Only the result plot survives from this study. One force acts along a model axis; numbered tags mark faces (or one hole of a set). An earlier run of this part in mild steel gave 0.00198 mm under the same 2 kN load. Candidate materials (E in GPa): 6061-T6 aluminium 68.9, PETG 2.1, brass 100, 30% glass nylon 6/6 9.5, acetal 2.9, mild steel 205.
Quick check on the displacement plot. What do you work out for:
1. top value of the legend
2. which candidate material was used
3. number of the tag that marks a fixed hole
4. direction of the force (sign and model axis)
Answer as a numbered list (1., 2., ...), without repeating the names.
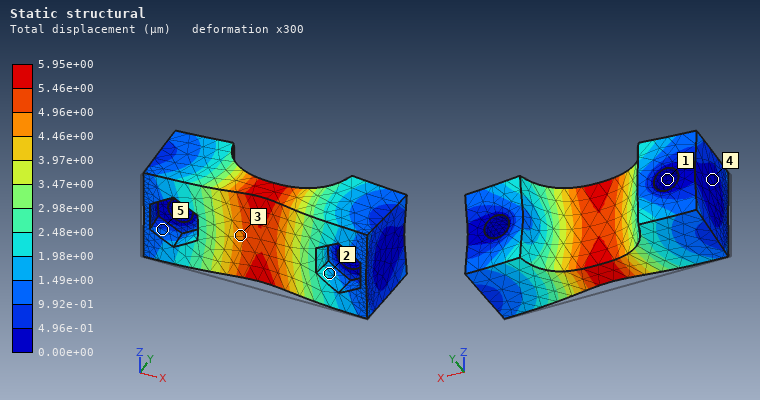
1. 5.95e+00 µm
2. 6061-T6 aluminium
3. 1
4. +Y
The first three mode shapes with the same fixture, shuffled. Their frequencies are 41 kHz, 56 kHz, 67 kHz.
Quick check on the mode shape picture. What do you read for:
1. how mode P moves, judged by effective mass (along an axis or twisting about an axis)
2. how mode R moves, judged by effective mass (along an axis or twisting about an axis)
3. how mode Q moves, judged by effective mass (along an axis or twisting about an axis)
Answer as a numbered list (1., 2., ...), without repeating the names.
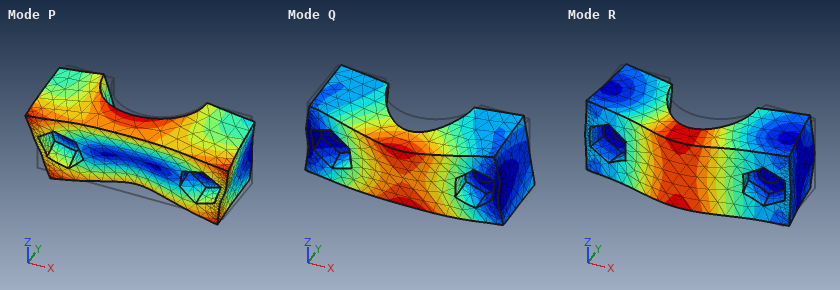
1. twisting about X
2. along Y
3. along Z
